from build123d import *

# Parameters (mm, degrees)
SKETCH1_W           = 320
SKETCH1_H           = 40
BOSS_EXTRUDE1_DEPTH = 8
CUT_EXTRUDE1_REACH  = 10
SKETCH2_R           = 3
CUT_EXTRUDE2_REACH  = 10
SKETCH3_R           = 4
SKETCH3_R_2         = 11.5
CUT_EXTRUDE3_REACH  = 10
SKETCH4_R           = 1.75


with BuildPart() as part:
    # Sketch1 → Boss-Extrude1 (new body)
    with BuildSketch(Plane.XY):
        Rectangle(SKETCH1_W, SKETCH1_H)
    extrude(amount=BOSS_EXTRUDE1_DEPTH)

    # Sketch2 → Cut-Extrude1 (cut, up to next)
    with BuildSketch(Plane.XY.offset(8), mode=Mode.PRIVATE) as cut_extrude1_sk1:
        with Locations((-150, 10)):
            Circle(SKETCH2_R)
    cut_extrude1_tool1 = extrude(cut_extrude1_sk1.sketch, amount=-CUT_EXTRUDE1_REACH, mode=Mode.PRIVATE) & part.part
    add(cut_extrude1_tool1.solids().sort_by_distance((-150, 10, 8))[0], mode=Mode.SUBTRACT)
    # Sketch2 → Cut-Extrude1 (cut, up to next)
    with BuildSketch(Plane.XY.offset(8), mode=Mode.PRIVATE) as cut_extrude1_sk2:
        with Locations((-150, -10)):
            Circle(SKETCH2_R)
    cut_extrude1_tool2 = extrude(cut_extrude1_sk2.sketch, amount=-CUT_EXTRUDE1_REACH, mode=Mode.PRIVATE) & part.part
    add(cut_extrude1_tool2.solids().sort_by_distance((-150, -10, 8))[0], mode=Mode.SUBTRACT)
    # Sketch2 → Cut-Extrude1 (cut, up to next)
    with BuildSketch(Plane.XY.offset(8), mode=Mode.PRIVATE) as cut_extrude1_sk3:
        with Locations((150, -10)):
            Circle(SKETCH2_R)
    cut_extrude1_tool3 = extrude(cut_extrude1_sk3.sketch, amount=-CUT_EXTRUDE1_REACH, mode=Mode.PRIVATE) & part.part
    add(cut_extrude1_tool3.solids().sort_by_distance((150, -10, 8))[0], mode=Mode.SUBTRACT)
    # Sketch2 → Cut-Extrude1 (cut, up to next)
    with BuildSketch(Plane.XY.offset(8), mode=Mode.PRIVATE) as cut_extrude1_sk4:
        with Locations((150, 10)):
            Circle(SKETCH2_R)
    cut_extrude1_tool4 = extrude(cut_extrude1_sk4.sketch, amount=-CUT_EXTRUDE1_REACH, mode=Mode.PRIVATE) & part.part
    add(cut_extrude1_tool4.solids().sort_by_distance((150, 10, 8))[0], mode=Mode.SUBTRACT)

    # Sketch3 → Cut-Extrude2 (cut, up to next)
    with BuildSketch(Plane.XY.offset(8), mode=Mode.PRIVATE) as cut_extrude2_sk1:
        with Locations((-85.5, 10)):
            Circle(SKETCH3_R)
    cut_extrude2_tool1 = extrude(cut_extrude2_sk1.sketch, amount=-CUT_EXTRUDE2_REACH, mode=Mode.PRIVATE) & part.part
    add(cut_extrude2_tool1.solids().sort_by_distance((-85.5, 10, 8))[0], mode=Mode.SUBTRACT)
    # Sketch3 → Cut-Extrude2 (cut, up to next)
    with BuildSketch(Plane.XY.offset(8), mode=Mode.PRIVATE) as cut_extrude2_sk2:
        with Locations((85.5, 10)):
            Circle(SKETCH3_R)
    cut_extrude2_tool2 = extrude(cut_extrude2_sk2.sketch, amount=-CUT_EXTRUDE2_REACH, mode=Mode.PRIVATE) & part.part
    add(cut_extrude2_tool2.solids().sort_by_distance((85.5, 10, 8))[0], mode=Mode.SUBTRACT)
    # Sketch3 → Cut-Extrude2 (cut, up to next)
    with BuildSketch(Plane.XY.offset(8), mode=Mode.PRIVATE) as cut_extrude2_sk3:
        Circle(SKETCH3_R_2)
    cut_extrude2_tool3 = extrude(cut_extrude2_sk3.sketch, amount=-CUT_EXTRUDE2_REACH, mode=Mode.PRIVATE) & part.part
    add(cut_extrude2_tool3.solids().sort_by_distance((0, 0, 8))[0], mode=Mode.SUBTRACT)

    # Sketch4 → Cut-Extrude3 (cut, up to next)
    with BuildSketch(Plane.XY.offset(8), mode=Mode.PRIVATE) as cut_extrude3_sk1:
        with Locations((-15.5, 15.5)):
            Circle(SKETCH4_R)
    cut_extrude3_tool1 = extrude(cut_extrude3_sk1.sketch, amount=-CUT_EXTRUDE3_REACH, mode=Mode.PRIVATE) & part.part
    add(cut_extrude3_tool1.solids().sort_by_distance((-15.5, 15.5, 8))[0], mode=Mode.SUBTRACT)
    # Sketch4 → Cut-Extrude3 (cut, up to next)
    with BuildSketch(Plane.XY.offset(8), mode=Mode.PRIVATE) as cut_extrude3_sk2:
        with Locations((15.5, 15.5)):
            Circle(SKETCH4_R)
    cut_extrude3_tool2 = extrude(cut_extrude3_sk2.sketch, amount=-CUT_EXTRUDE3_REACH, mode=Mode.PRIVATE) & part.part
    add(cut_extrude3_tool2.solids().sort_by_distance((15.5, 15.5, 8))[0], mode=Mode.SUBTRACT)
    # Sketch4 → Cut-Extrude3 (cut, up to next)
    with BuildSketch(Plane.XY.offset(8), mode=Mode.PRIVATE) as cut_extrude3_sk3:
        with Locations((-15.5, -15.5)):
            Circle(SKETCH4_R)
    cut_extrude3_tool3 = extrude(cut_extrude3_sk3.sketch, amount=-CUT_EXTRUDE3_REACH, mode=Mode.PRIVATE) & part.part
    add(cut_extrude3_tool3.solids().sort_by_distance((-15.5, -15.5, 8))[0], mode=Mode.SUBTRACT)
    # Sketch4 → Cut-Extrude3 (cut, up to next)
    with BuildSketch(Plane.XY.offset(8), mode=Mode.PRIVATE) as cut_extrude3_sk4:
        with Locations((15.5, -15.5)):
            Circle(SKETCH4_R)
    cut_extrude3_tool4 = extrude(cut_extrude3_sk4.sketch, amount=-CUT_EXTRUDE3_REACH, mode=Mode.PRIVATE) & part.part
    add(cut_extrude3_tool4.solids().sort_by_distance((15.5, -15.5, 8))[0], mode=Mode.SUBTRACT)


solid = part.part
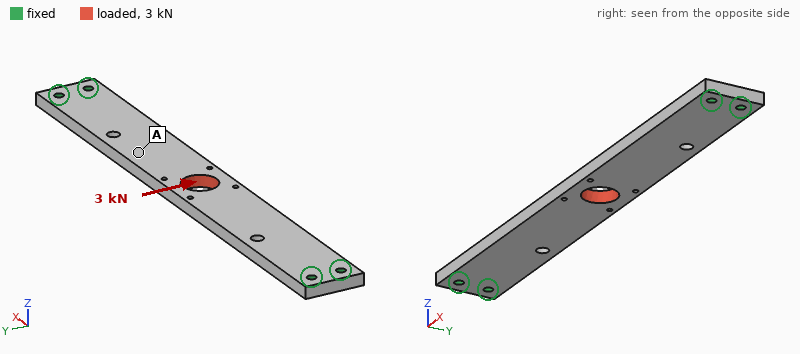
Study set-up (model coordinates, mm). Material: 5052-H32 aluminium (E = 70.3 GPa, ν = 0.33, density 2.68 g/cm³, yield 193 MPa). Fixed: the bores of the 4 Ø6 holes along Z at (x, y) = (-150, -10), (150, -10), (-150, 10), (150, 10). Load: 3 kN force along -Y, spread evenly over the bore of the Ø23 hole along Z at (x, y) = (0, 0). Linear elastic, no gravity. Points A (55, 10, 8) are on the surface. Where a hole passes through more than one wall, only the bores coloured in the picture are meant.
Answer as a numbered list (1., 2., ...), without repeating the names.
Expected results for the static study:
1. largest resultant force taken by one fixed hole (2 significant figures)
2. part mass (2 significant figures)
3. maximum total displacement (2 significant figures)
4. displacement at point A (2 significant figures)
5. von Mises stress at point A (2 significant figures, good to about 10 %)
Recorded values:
1. 4.7 kN
2. 260 g
3. 0.19 mm
4. 0.13 mm
5. 12 MPa
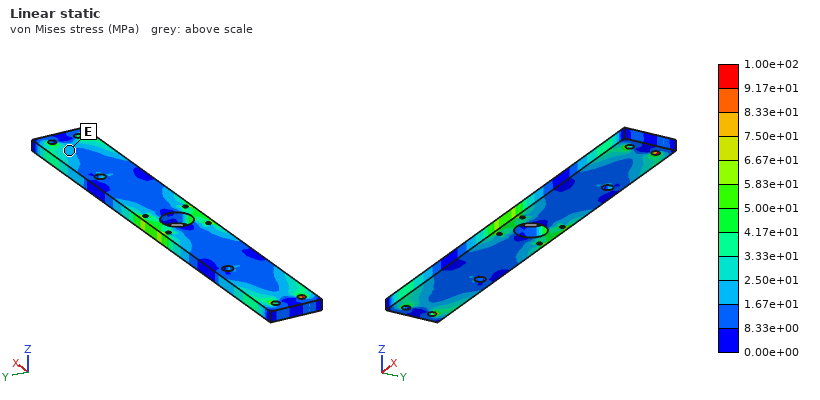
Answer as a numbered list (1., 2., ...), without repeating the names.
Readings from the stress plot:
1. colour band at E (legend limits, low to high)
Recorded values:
1. 1.67e+01 to 2.50e+01 MPa
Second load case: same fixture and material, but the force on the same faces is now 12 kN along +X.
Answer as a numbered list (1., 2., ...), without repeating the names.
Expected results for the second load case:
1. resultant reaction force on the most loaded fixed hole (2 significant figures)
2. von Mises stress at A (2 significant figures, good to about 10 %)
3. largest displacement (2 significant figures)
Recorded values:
1. 3.1 kN
2. 18 MPa
3. 43 µm
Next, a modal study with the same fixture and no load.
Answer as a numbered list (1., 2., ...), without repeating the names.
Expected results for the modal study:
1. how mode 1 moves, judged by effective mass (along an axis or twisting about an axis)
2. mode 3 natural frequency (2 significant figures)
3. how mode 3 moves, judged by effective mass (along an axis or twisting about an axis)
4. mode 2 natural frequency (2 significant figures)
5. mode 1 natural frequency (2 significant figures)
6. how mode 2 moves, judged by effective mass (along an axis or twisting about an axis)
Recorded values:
1. along Z
2. 2100 Hz
3. twisting about X
4. 1300 Hz
5. 470 Hz
6. twisting about Y
